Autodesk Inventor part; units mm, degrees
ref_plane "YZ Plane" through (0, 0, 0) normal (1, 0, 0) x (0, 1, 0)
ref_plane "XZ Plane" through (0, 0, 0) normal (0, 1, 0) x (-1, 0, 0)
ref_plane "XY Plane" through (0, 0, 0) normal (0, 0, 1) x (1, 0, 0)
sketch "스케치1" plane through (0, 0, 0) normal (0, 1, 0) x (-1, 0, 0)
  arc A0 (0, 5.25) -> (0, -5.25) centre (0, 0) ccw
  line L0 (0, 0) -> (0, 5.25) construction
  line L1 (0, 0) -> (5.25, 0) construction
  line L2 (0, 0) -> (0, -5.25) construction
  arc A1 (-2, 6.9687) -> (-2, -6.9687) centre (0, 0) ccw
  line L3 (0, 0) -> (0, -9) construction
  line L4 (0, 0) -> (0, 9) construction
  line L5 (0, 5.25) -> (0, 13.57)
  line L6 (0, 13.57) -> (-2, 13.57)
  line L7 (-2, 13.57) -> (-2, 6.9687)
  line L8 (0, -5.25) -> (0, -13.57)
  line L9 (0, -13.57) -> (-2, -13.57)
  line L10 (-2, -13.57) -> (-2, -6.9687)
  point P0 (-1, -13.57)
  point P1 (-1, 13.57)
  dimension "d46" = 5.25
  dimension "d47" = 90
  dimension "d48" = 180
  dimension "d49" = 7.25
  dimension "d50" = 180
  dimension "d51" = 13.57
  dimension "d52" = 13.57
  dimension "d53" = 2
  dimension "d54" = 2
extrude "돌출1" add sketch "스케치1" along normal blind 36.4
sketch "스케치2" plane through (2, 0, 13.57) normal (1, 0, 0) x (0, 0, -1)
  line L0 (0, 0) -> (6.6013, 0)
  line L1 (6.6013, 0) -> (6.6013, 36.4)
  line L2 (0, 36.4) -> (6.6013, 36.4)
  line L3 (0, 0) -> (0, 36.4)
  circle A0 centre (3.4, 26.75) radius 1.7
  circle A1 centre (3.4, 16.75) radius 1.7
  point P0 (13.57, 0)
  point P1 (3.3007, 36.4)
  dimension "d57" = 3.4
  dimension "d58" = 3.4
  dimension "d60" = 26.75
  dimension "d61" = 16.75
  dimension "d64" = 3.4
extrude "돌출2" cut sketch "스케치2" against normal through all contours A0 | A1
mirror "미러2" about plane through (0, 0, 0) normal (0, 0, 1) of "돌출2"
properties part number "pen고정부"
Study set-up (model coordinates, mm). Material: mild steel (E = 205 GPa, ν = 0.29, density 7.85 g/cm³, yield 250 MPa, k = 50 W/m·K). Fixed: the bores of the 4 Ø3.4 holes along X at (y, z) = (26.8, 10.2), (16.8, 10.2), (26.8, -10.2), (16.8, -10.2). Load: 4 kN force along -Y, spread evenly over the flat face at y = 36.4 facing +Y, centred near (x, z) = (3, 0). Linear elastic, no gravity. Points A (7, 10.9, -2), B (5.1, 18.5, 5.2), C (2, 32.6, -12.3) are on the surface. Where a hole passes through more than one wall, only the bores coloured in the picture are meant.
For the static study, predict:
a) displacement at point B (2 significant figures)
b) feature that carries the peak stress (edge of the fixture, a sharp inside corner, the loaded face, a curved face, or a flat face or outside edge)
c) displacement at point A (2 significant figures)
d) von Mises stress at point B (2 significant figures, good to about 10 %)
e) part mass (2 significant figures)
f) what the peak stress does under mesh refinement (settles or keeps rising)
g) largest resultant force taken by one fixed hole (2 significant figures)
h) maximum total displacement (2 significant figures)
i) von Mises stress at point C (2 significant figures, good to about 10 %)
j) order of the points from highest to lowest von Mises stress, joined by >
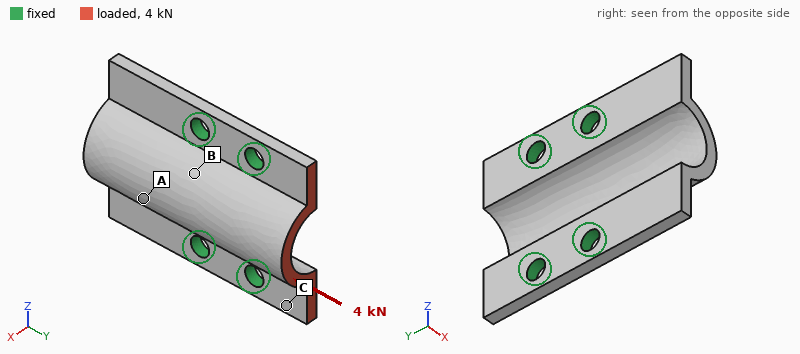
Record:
3.7 µm
edge of the fixture
6.9 µm
39 MPa
18 g
keeps rising
1.5 kN
15 µm
70 MPa
C > B > A
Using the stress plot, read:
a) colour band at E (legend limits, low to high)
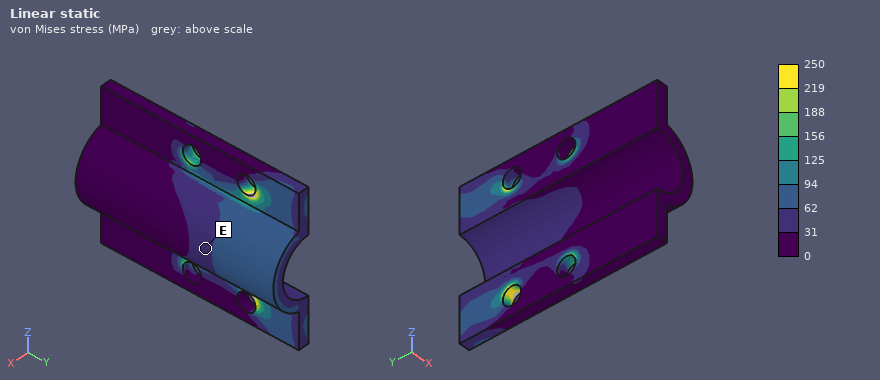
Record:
31 to 62 MPa
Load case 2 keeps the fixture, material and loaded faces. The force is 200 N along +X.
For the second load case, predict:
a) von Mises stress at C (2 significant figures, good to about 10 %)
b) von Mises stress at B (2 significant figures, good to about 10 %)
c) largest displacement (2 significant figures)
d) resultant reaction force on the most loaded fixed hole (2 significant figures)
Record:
22 MPa
7.1 MPa
6.2 µm
180 N
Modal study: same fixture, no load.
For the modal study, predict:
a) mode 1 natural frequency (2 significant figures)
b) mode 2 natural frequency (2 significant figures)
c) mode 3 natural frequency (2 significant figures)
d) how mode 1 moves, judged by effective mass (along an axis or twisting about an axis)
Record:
11 kHz
13 kHz
20 kHz
along X
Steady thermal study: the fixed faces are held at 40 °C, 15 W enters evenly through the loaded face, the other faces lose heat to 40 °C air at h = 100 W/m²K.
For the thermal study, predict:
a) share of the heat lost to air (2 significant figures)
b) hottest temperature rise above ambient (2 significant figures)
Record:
15 %
51 K
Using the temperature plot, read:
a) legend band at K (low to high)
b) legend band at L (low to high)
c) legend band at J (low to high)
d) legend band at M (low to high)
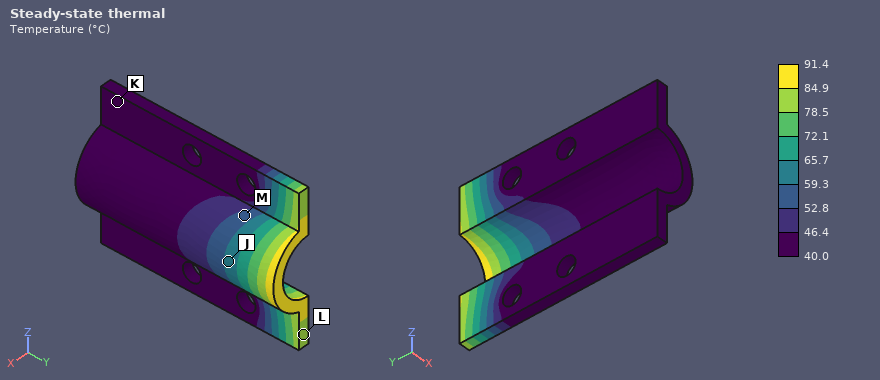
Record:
40.0 to 46.4 °C
78.5 to 84.9 °C
59.3 to 65.7 °C
52.8 to 59.3 °C
